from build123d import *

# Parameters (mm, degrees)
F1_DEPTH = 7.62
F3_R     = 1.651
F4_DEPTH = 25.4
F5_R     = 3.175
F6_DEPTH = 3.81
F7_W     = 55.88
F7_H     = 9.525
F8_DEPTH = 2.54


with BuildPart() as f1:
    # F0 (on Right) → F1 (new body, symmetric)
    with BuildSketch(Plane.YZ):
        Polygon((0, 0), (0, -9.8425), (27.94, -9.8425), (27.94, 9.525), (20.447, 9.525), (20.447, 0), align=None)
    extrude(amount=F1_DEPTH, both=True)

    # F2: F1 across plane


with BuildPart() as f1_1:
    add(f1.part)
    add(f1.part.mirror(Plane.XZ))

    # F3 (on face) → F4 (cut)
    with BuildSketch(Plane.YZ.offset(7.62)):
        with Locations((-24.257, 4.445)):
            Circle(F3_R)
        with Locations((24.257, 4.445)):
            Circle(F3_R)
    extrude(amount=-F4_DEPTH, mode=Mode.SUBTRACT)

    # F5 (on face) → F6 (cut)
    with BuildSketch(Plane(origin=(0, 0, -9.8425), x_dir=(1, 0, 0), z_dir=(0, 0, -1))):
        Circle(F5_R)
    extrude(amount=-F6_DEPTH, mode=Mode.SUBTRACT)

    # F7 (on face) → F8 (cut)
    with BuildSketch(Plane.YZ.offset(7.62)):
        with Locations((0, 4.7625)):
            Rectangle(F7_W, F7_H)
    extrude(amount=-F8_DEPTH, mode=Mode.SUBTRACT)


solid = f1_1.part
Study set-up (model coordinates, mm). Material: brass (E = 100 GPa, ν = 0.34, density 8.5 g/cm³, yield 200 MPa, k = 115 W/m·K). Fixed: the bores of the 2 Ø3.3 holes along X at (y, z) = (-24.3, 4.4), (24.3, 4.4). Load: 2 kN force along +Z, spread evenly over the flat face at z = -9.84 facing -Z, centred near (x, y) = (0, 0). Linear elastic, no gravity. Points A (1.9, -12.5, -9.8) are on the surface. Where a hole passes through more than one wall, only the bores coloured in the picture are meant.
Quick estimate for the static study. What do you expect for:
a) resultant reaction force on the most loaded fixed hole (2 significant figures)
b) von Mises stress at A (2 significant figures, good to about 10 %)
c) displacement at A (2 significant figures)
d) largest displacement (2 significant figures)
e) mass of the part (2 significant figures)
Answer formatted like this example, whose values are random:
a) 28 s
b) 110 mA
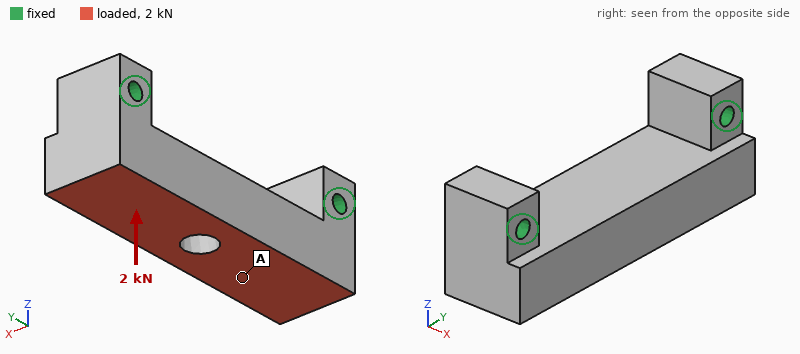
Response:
a) 1.2 kN
b) 8.0 MPa
c) 6.4 µm
d) 10 µm
e) 84 g
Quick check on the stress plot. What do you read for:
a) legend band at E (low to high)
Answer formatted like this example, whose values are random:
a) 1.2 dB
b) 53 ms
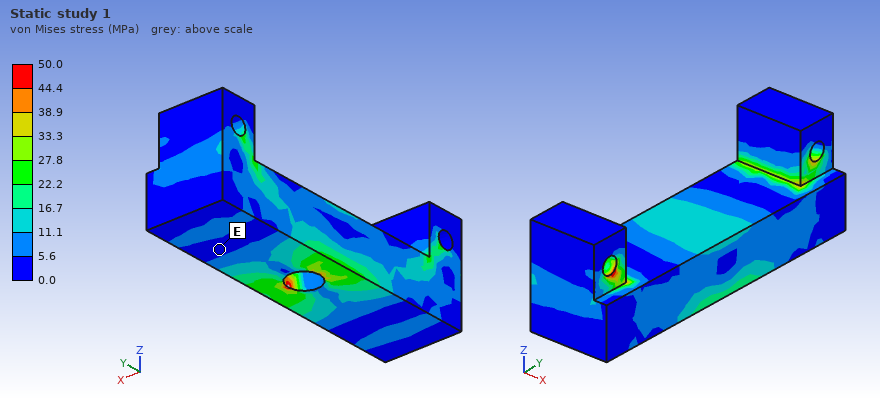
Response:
a) 0.0 to 5.6 MPa
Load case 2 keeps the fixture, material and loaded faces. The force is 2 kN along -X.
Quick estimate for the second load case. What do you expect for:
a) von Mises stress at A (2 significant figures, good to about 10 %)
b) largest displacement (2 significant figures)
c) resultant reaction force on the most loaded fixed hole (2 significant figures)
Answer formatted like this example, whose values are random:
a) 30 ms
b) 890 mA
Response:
a) 17 MPa
b) 19 µm
c) 1.0 kN
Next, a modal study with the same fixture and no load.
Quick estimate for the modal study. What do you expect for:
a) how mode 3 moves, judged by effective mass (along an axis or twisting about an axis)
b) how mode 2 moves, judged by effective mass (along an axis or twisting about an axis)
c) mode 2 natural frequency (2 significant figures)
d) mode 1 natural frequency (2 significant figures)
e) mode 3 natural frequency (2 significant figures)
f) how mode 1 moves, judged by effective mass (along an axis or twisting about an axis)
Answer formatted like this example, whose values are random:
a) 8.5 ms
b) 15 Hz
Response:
a) along Y
b) along Z
c) 10000 Hz
d) 8900 Hz
e) 12 kHz
f) along X
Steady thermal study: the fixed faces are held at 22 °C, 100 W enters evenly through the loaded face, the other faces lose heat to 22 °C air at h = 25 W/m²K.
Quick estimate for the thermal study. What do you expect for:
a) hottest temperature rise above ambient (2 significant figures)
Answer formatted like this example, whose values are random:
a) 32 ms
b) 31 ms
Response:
a) 57 K
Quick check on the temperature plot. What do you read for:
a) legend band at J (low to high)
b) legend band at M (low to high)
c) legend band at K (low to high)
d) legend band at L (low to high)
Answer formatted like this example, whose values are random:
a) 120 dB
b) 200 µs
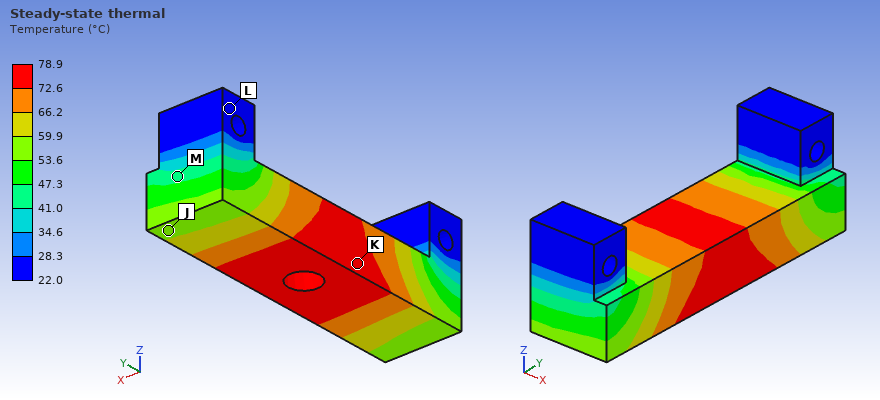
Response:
a) 53.6 to 59.9 °C
b) 41.0 to 47.3 °C
c) 72.6 to 78.9 °C
d) 22.0 to 28.3 °C
